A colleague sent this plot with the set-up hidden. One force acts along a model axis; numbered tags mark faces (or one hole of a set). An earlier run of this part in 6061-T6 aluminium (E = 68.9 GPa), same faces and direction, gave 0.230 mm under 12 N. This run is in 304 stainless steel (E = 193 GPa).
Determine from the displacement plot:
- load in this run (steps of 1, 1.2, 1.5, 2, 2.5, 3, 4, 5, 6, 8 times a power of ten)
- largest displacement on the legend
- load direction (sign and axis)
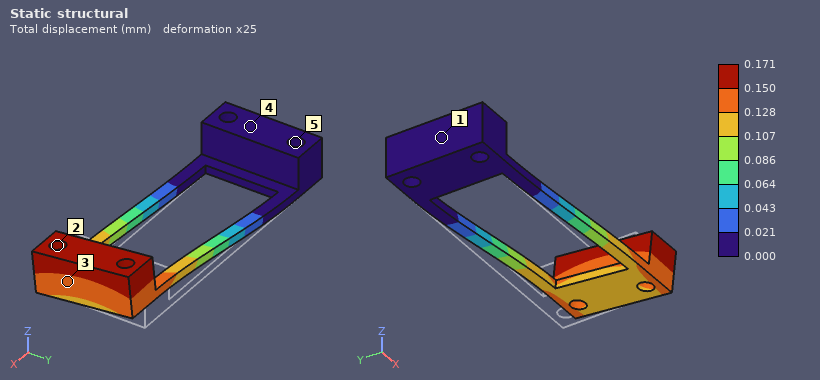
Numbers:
25 N
0.171 mm
-Y
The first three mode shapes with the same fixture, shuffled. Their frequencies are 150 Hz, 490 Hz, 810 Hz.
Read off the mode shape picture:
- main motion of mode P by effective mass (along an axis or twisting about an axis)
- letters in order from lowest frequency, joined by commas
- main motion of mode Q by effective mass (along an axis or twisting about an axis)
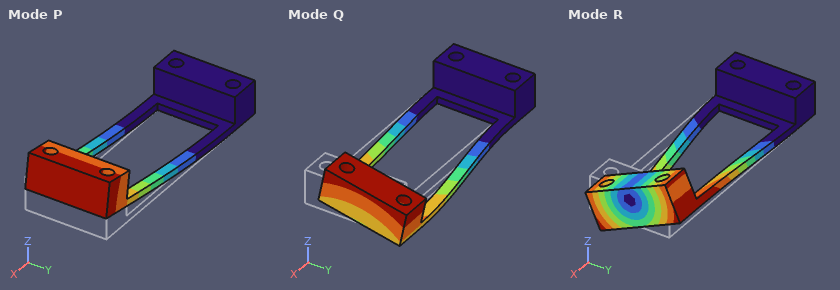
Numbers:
along Z
P, Q, R
along Y
